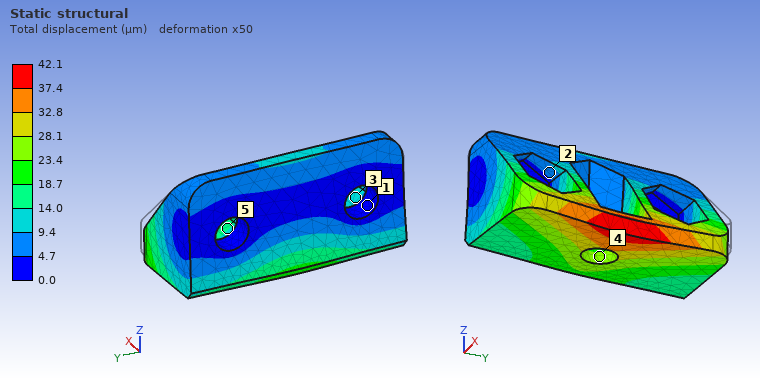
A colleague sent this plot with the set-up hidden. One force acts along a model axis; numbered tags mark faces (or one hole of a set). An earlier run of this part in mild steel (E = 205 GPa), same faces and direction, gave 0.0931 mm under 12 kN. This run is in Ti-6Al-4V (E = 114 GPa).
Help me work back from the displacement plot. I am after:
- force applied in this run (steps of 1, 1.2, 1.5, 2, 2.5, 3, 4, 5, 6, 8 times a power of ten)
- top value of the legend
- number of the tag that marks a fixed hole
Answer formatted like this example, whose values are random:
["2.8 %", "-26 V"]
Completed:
["3 kN", "42.1 µm", "1"]
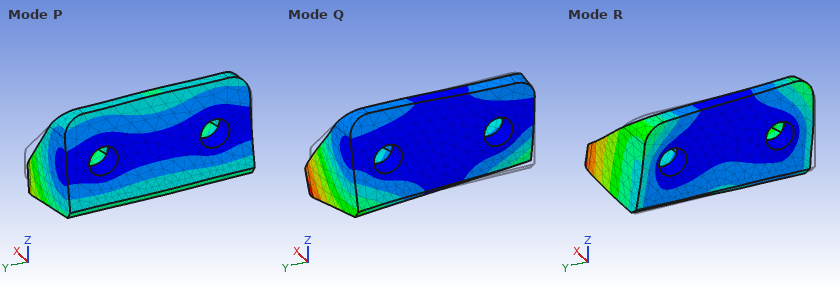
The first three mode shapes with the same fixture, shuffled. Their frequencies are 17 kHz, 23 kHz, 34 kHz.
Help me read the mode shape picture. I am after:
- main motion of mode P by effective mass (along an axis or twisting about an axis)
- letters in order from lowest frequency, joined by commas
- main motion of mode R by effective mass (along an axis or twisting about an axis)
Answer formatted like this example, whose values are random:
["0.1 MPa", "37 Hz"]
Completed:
["along Z", "P, Q, R", "along Y"]
